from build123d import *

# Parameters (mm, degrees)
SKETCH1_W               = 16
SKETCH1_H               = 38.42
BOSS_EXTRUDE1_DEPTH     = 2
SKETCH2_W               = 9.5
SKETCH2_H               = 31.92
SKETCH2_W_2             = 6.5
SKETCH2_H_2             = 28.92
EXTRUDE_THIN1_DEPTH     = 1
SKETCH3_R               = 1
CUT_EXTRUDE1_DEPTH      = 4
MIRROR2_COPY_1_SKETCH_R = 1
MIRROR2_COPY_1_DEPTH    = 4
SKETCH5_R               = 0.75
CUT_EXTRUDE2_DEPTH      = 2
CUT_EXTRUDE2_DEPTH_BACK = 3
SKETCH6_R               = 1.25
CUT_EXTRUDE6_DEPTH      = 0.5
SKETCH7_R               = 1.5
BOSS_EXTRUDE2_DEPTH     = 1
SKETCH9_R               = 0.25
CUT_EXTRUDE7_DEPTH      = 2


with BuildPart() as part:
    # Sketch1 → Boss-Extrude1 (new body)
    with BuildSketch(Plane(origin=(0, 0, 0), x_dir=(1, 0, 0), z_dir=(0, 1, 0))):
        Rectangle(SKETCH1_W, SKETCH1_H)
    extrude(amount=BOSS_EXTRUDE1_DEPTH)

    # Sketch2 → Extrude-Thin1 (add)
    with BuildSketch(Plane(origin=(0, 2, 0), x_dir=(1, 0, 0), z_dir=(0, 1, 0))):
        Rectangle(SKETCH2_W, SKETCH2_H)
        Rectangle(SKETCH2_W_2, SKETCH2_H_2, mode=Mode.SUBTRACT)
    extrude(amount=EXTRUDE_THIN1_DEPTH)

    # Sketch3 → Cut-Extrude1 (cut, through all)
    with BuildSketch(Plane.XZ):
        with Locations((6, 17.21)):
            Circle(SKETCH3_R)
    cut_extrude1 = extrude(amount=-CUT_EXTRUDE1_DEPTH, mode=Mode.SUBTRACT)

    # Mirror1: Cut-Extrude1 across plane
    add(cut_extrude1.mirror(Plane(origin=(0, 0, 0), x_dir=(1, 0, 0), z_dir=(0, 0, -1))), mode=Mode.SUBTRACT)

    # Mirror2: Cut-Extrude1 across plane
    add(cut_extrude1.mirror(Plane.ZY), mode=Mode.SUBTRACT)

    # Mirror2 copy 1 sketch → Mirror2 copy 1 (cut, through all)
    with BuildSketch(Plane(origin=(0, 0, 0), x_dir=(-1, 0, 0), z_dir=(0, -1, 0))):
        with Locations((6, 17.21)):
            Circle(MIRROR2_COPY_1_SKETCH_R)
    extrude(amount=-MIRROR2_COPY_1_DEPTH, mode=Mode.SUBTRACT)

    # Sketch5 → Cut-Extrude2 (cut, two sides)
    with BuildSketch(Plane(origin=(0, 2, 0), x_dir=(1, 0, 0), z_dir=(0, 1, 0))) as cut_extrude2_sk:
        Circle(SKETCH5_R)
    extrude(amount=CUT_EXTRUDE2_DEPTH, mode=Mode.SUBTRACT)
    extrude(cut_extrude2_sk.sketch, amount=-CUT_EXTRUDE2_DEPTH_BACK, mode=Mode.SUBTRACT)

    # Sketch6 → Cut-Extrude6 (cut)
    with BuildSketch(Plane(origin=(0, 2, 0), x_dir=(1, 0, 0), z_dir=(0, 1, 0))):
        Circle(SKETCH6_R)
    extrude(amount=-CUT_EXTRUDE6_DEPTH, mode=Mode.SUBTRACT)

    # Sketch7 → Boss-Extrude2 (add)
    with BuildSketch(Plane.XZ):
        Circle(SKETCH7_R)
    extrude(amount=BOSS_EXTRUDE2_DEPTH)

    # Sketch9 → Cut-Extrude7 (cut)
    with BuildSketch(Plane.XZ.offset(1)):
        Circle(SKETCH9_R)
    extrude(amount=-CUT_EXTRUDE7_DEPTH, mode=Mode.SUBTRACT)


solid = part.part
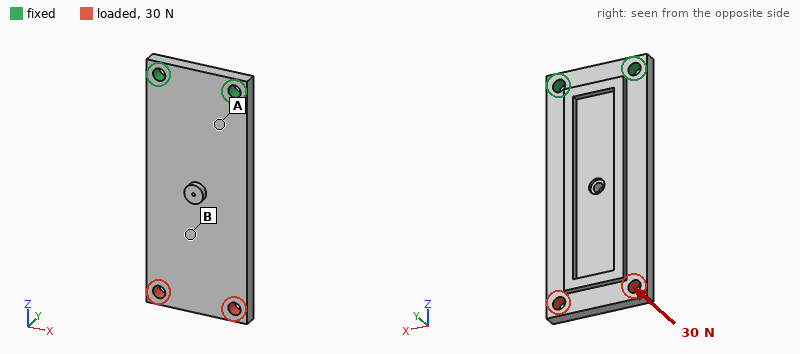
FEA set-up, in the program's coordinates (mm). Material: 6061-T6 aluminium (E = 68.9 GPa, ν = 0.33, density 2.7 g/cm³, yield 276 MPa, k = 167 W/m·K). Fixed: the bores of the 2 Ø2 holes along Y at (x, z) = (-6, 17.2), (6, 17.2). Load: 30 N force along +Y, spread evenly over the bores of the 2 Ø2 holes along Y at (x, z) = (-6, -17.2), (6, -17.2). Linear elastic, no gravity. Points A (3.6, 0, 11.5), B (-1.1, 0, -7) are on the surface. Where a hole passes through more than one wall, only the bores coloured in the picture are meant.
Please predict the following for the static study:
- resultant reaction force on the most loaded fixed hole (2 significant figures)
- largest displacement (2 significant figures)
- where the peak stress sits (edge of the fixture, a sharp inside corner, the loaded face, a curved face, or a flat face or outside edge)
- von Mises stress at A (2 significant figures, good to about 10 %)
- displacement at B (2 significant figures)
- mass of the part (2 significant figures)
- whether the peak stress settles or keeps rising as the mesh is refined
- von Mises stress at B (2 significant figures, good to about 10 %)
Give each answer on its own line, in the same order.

15 N
0.43 mm
edge of the fixture
58 MPa
0.23 mm
3.6 g
keeps rising
20 MPa
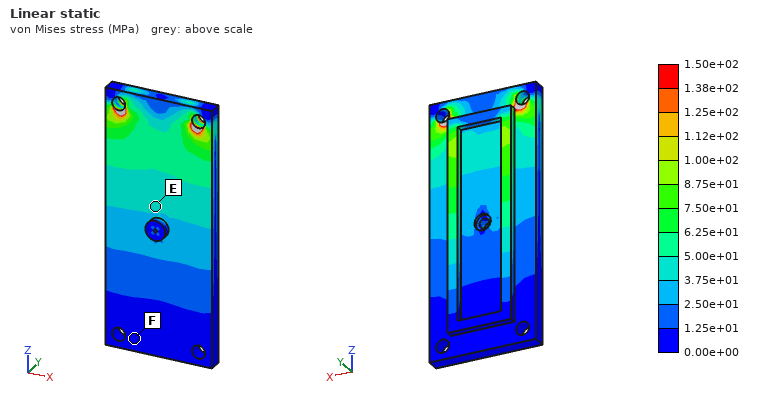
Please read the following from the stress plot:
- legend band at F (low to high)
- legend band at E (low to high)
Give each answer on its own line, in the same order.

0.00e+00 to 1.25e+01 MPa
3.75e+01 to 5.00e+01 MPa
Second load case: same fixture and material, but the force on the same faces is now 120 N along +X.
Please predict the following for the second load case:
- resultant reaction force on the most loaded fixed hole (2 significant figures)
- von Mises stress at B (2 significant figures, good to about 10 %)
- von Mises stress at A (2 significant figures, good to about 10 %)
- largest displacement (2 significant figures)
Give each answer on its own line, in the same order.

340 N
10 MPa
19 MPa
43 µm
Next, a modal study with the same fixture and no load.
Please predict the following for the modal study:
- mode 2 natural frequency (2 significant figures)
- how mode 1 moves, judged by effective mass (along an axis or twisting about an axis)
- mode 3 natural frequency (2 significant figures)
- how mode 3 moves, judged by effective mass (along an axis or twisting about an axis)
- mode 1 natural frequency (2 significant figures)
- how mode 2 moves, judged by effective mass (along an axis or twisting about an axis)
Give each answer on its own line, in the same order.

6200 Hz
along Y
8700 Hz
along X
1400 Hz
twisting about Z
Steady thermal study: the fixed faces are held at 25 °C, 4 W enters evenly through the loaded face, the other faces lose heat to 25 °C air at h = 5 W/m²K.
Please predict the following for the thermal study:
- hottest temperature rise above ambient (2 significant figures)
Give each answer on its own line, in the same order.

26 K
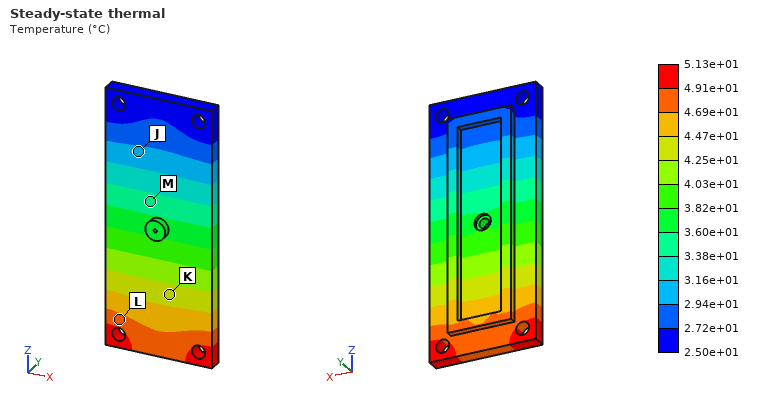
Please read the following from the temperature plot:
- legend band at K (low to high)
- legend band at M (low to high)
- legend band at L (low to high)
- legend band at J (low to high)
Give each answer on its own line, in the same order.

4.25e+01 to 4.47e+01 °C
3.38e+01 to 3.60e+01 °C
4.69e+01 to 4.91e+01 °C
2.94e+01 to 3.16e+01 °C
